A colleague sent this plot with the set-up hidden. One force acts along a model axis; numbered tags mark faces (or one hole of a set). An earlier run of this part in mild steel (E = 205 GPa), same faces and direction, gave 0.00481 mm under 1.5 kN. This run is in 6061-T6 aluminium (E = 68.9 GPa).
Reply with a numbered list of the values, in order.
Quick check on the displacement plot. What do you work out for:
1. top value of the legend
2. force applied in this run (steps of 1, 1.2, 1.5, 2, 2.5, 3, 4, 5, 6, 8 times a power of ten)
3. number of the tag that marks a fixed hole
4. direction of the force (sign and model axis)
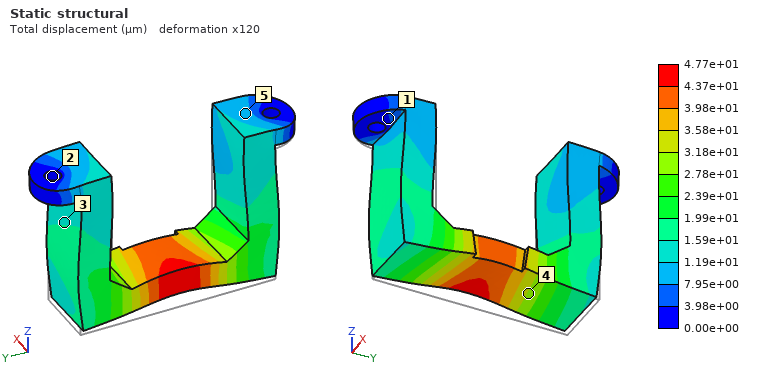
1. 4.77e+01 µm
2. 5 kN
3. 2
4. +Z
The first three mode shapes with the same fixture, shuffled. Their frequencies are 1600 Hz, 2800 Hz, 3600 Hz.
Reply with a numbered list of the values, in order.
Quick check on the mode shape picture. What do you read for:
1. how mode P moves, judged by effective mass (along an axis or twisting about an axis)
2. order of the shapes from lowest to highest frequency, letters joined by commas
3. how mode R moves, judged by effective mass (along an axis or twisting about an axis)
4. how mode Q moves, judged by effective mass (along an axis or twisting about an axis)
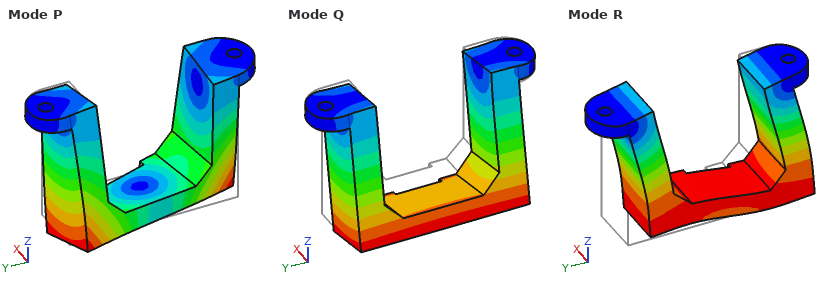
1. twisting about Z
2. Q, R, P
3. along Y
4. along X
